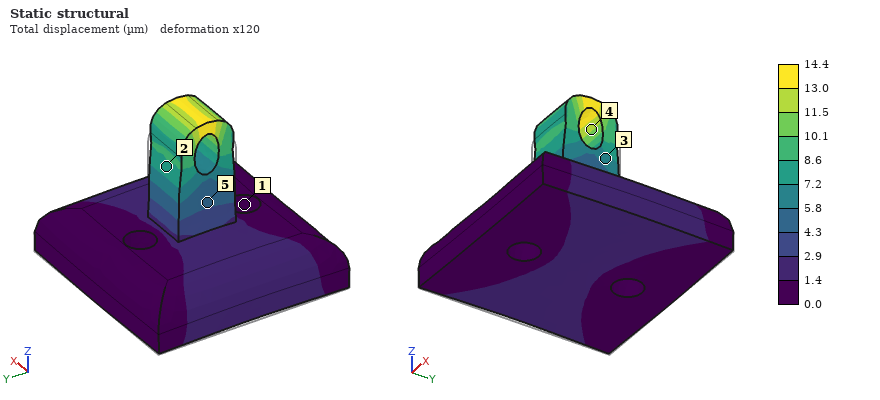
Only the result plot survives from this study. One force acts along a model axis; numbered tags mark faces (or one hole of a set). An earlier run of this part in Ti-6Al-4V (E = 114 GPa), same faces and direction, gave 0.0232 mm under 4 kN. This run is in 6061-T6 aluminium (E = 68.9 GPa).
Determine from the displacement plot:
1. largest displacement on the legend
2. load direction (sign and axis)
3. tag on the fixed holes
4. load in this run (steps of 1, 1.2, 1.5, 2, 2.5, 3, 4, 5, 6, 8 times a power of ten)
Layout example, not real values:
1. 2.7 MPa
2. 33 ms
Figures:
1. 14.4 µm
2. +Z
3. 1
4. 1.5 kN
